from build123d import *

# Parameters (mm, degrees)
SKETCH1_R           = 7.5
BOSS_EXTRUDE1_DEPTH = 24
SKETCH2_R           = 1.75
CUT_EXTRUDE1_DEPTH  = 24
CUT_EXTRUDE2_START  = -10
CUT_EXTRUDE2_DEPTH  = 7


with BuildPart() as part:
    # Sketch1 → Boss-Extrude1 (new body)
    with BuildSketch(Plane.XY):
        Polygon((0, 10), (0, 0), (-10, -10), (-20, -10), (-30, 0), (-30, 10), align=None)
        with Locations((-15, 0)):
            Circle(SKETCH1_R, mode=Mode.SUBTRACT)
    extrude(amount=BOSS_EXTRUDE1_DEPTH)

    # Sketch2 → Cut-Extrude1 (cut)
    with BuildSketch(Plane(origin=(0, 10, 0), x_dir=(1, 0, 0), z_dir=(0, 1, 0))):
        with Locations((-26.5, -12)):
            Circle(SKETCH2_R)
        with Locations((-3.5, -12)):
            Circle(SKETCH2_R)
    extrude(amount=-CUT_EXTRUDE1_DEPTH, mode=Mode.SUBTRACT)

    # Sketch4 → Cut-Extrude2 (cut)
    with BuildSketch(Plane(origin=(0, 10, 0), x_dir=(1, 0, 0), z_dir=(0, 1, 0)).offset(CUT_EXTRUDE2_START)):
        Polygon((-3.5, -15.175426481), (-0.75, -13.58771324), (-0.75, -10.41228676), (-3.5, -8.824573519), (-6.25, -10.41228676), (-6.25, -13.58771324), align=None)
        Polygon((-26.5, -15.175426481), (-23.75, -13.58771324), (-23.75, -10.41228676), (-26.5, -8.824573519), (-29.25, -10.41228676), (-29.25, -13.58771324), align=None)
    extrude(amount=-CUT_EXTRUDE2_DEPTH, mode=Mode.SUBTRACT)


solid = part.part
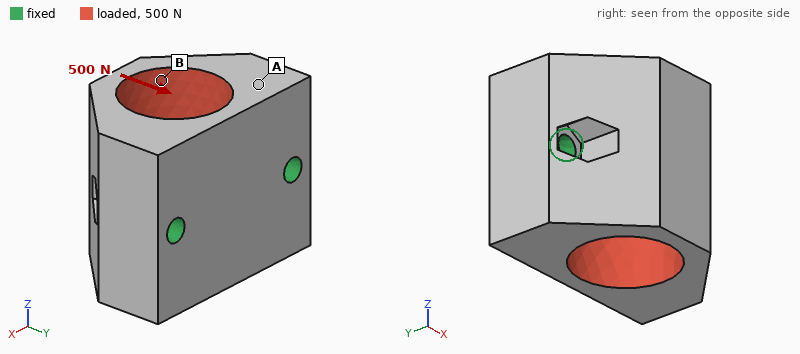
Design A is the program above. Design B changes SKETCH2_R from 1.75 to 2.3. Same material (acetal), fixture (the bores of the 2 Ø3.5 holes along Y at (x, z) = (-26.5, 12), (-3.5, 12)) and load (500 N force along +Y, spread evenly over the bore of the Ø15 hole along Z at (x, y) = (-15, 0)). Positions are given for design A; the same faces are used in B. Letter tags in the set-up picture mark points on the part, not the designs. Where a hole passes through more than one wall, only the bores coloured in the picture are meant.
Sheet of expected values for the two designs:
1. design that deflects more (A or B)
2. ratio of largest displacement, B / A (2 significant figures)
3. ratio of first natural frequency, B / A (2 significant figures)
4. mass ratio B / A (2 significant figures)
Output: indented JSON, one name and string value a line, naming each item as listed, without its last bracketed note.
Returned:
{
  "design that deflects more": "A",
  "ratio of largest displacement, B / A": "0.89",
  "ratio of first natural frequency, B / A": "1.1",
  "mass ratio B / A": "0.98"
}
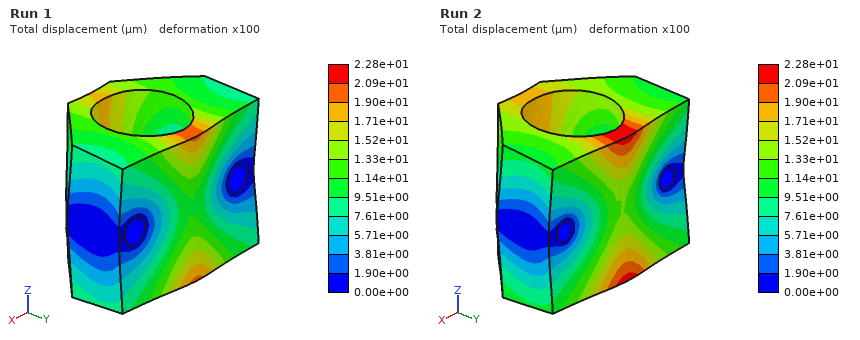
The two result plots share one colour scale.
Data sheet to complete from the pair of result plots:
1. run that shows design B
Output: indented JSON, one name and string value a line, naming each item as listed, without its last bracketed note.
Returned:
{
  "run that shows design B": "Run 1"
}
